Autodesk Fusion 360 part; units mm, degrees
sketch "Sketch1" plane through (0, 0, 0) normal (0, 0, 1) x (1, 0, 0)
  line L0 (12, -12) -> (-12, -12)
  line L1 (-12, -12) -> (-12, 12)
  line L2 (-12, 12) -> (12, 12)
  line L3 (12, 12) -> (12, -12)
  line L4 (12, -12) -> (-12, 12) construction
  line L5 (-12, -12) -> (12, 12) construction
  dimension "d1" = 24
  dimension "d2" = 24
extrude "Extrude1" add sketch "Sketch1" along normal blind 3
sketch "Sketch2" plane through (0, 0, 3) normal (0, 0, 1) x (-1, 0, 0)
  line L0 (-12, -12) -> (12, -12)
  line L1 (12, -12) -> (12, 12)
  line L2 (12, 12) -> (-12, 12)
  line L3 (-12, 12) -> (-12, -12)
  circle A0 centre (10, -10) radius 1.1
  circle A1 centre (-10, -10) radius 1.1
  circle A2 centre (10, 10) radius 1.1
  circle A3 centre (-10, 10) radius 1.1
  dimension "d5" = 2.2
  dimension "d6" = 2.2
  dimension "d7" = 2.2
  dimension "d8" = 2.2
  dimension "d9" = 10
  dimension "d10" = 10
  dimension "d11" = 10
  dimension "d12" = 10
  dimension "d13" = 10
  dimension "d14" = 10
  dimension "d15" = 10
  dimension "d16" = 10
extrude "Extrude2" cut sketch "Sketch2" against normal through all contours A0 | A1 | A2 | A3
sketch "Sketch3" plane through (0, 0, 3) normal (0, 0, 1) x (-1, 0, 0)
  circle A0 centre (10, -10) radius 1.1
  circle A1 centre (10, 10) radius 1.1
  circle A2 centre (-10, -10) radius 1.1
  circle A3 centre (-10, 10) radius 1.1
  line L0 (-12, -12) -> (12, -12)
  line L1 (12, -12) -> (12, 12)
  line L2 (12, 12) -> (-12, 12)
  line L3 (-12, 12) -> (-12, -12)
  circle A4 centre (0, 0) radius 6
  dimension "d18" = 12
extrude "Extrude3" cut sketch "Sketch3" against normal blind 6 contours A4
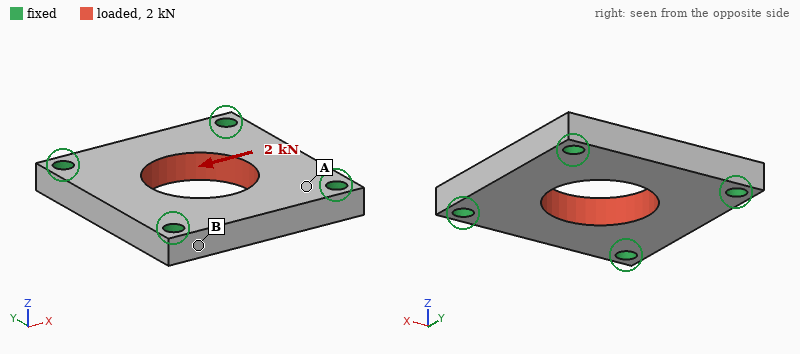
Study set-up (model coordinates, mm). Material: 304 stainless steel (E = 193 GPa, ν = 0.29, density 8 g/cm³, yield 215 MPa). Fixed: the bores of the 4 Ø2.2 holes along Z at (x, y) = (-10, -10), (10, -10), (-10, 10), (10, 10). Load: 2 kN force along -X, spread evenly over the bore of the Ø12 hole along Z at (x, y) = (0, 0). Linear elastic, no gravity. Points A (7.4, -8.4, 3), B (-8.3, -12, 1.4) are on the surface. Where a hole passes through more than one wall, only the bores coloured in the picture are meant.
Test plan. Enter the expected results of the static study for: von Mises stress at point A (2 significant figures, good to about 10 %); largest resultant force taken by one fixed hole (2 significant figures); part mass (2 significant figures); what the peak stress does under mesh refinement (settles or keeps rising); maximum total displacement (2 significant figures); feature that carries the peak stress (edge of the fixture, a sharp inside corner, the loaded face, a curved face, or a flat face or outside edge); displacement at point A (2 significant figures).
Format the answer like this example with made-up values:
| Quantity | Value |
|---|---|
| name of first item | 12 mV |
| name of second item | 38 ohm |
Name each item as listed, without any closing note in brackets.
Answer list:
| Quantity | Value |
|---|---|
| von Mises stress at point A | 31 MPa |
| largest resultant force taken by one fixed hole | 540 N |
| part mass | 11 g |
| what the peak stress does under mesh refinement | keeps rising |
| maximum total displacement | 2.5 µm |
| feature that carries the peak stress | edge of the fixture |
| displacement at point A | 0.56 µm |
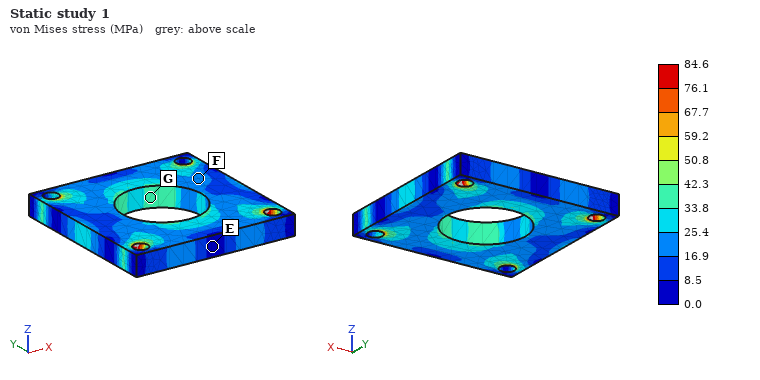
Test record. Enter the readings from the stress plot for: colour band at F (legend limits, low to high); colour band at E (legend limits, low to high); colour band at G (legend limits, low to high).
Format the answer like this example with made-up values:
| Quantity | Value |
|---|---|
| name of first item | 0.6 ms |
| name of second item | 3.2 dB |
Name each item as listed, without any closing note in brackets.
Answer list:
| Quantity | Value |
|---|---|
| colour band at F | 16.9 to 25.4 MPa |
| colour band at E | 0.0 to 8.5 MPa |
| colour band at G | 33.8 to 42.3 MPa |
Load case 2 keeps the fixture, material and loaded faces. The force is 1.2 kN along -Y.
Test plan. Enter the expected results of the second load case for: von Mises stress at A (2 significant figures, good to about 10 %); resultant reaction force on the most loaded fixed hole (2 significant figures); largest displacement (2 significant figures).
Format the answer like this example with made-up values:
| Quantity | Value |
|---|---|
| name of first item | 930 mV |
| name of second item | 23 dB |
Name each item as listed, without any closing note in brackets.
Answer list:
| Quantity | Value |
|---|---|
| von Mises stress at A | 18 MPa |
| resultant reaction force on the most loaded fixed hole | 320 N |
| largest displacement | 1.5 µm |
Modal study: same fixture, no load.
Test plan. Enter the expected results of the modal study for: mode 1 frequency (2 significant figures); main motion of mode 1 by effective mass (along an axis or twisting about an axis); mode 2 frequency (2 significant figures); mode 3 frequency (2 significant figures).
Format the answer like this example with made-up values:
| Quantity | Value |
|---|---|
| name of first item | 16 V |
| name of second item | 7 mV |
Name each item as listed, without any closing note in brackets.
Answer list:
| Quantity | Value |
|---|---|
| mode 1 frequency | 29 kHz |
| main motion of mode 1 by effective mass | along Z |
| mode 2 frequency | 37 kHz |
| mode 3 frequency | 37 kHz |
